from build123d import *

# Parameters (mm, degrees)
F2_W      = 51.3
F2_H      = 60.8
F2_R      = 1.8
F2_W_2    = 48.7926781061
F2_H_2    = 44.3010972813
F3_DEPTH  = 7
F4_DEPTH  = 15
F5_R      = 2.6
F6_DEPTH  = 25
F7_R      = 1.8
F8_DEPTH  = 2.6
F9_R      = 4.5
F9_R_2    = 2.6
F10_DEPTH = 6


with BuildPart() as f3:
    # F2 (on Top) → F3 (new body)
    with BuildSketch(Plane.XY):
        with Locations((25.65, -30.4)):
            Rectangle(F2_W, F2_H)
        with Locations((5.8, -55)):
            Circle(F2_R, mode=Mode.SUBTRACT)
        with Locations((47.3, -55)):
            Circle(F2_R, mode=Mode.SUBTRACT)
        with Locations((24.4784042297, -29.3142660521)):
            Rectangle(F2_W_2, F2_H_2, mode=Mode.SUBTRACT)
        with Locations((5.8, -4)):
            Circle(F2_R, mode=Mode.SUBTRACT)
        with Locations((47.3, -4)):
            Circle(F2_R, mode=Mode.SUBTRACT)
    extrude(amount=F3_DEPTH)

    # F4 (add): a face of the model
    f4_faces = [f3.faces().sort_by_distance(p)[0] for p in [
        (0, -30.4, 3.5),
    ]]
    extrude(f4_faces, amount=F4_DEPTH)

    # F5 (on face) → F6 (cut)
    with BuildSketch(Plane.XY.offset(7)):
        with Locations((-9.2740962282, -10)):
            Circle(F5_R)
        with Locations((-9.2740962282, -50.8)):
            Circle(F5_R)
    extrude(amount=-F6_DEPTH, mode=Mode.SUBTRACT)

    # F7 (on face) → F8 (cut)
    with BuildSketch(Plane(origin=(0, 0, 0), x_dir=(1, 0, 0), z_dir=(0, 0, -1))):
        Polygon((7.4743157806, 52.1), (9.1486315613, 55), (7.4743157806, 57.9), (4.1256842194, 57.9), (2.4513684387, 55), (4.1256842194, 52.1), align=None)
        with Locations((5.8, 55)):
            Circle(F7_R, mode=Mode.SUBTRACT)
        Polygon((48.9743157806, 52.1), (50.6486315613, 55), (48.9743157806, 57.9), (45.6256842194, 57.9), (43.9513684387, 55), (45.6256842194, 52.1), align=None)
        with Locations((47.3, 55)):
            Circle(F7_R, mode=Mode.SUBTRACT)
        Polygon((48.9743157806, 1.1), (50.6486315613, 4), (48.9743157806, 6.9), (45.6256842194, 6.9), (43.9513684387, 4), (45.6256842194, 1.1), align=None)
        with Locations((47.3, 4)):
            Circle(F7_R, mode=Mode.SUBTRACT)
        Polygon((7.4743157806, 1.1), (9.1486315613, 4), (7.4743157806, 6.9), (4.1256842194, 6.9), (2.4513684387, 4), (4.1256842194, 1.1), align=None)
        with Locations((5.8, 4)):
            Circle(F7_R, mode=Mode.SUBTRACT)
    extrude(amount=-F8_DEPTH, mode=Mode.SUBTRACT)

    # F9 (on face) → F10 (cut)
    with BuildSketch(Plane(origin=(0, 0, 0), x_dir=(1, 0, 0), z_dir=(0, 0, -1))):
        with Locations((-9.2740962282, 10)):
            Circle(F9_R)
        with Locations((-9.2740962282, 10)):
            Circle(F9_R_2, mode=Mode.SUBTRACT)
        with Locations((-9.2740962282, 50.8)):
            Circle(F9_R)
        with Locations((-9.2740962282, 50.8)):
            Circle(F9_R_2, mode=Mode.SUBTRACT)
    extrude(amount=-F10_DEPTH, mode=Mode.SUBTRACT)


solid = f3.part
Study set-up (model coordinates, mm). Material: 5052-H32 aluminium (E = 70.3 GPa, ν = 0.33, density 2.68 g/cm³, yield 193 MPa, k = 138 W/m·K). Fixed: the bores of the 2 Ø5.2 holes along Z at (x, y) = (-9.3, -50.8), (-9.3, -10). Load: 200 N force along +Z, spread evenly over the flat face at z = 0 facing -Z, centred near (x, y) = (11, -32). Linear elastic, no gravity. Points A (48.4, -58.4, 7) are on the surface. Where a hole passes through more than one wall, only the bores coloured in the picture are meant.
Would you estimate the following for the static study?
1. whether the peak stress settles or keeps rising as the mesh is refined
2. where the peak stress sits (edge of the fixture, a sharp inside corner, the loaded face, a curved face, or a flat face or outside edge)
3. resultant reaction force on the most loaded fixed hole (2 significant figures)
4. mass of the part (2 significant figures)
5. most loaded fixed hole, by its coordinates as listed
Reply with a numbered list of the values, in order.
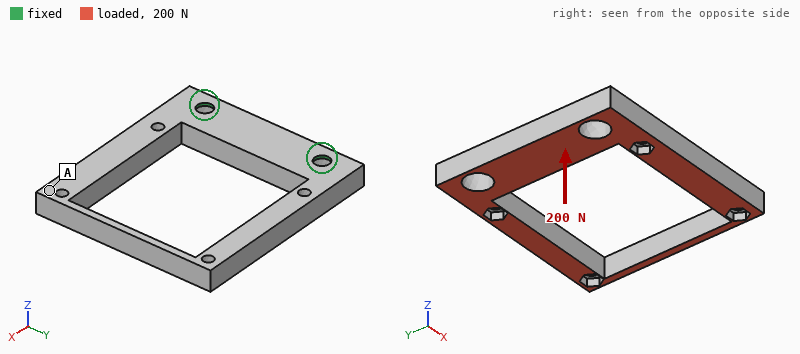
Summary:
1. keeps rising
2. edge of the fixture
3. 110 N
4. 32 g
5. (-9.3, -50.8)
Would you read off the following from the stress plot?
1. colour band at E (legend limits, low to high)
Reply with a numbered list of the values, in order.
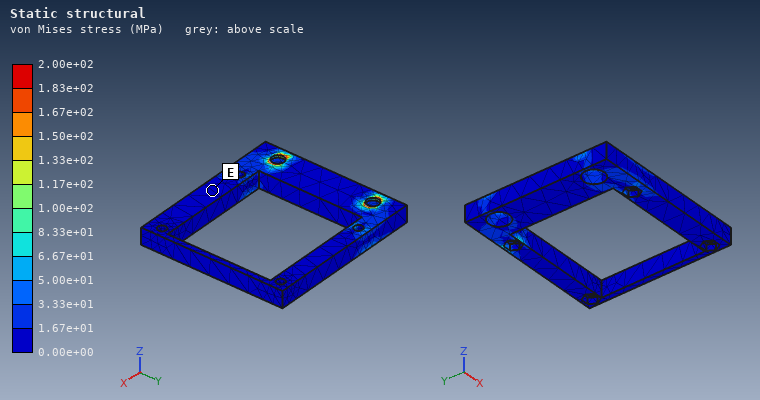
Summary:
1. 0.00e+00 to 1.67e+01 MPa
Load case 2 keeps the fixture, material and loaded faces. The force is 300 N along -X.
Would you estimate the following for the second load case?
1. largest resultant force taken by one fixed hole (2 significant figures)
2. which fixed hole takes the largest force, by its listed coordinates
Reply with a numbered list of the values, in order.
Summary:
1. 160 N
2. (-9.3, -50.8)
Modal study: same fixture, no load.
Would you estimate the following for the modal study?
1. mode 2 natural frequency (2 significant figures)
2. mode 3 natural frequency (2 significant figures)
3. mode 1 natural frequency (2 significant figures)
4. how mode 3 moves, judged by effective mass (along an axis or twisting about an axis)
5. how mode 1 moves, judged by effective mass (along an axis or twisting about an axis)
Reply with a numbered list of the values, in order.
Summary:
1. 1700 Hz
2. 1700 Hz
3. 790 Hz
4. along Y
5. along Z
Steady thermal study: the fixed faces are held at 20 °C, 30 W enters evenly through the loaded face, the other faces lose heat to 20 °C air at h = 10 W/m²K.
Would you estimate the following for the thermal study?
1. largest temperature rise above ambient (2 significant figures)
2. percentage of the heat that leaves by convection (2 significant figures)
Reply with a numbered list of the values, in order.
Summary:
1. 54 K
2. 5.9 %
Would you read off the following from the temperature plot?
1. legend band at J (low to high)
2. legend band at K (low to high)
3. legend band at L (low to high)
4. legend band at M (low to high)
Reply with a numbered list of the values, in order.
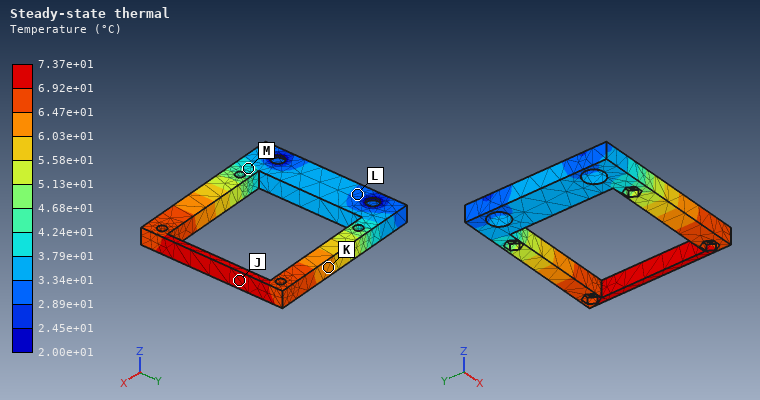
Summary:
1. 6.92e+01 to 7.37e+01 °C
2. 6.03e+01 to 6.47e+01 °C
3. 2.89e+01 to 3.34e+01 °C
4. 3.79e+01 to 4.24e+01 °C
